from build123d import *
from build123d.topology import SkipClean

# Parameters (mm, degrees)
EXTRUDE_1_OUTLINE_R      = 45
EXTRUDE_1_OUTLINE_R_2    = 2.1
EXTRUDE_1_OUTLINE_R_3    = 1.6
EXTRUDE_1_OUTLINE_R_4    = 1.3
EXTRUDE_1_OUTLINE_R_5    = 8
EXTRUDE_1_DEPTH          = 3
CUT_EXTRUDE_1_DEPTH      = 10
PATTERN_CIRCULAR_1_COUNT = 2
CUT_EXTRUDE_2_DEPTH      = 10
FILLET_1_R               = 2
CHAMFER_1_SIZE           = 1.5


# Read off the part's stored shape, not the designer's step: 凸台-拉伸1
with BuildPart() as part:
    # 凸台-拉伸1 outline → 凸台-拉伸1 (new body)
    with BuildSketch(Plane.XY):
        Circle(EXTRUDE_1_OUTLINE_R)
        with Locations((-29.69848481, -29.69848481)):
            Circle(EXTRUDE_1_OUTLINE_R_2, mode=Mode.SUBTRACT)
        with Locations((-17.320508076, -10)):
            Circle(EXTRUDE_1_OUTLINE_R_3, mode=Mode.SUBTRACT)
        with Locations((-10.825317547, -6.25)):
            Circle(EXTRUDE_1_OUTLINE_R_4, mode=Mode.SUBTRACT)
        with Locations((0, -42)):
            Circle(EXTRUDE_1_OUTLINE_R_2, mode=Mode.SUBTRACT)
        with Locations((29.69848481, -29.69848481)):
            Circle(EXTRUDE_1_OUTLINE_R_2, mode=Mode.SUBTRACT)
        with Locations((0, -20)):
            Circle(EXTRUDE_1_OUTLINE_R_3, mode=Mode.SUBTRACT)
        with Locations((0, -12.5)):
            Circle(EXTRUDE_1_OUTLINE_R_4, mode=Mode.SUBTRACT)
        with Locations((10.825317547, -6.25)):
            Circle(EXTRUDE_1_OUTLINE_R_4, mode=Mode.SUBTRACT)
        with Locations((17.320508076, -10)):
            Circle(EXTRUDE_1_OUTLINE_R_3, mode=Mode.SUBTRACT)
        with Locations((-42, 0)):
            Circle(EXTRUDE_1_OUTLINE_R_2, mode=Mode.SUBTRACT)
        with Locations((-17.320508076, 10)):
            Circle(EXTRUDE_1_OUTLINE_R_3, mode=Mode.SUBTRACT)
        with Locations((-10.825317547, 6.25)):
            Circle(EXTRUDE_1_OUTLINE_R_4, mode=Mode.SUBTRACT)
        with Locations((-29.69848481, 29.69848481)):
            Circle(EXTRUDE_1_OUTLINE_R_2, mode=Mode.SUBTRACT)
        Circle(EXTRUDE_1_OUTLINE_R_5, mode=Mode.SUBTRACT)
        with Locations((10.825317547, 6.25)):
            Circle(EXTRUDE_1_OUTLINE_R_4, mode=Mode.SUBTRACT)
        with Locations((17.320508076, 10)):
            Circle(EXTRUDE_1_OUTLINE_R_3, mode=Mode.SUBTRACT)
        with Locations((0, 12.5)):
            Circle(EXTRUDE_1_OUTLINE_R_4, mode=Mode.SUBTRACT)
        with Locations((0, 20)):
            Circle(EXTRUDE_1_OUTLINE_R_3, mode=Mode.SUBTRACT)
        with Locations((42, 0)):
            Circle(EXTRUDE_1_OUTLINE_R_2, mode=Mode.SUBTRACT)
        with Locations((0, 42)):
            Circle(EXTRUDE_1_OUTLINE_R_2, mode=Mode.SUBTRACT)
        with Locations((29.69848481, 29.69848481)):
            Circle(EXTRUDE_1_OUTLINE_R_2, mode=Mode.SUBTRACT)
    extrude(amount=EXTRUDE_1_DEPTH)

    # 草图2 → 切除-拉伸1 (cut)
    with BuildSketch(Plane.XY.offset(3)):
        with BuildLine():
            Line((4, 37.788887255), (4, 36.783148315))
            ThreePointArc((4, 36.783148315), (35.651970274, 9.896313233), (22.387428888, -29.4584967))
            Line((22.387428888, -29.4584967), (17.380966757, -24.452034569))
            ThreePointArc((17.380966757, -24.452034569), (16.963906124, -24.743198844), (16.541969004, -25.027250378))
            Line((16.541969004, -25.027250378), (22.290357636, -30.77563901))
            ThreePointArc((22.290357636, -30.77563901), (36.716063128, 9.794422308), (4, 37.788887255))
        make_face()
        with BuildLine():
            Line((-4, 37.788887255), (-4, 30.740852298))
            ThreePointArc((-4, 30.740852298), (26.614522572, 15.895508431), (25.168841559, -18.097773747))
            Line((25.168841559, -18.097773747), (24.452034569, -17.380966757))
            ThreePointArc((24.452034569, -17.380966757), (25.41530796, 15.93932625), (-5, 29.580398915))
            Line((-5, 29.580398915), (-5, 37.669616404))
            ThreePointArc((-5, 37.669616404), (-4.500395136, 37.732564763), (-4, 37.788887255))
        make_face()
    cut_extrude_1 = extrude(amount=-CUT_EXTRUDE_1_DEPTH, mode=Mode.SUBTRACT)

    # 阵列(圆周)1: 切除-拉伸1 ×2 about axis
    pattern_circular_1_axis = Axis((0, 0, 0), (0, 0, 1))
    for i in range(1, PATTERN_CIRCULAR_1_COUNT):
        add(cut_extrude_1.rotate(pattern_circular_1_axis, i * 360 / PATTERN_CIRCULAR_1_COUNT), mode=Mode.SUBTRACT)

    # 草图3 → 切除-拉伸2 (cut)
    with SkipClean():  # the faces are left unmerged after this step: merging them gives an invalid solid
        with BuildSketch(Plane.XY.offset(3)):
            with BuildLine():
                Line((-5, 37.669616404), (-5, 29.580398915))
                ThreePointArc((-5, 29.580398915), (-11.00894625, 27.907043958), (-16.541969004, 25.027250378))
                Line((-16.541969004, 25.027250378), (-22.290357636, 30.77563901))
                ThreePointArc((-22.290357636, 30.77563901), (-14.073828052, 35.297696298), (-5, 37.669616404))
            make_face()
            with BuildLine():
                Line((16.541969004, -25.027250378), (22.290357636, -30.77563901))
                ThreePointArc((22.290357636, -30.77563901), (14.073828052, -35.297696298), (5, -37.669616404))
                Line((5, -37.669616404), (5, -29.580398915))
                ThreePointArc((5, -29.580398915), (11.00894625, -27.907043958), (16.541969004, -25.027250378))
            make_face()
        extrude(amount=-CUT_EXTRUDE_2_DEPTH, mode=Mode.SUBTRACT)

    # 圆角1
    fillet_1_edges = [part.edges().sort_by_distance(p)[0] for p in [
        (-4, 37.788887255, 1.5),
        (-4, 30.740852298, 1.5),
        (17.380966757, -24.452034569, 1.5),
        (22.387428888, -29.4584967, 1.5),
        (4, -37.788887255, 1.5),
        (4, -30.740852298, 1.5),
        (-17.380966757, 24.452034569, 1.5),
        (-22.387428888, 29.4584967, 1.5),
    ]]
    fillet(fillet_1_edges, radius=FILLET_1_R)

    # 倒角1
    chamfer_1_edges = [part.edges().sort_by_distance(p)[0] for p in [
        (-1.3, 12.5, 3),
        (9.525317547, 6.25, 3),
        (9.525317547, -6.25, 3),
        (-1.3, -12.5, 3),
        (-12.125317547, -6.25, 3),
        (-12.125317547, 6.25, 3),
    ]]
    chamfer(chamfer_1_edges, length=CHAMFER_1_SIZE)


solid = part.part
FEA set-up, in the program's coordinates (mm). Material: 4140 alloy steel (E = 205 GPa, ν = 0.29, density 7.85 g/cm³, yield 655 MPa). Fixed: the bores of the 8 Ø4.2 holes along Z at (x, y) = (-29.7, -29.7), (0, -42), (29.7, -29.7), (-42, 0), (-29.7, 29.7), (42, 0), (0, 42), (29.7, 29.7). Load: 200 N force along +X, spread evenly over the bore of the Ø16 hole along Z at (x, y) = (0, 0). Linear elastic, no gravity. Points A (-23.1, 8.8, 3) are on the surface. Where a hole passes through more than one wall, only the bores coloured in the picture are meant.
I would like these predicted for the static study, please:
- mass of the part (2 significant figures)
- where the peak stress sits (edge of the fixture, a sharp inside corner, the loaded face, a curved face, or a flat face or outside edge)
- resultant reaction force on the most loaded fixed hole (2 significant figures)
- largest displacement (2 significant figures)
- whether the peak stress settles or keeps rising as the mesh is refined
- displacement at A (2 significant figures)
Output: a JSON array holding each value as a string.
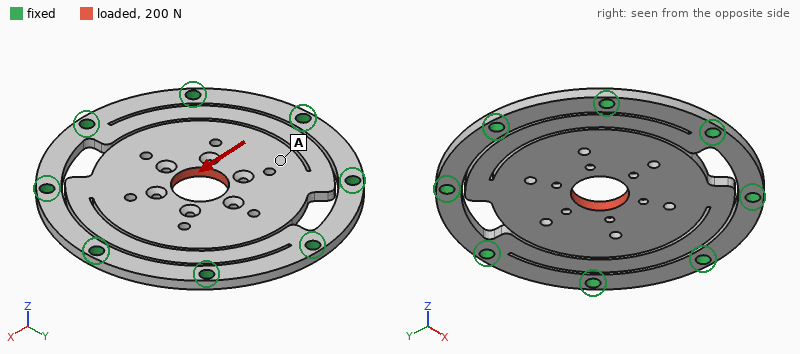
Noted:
["130 g", "a sharp inside corner", "140 N", "0.28 mm", "keeps rising", "0.28 mm"]
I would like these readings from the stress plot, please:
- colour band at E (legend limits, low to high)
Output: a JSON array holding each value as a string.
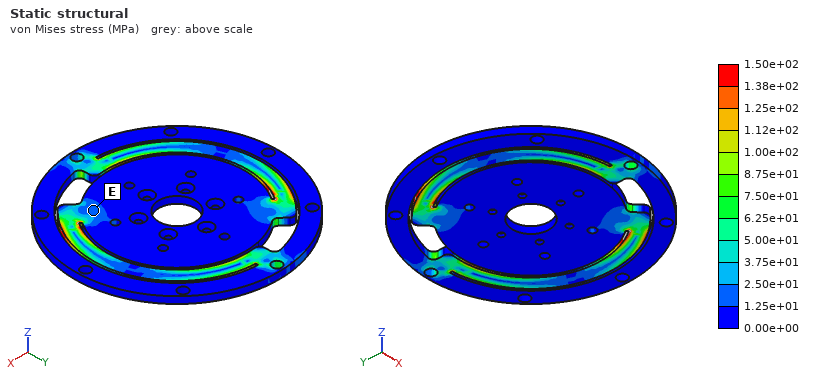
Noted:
["1.25e+01 to 2.50e+01 MPa"]
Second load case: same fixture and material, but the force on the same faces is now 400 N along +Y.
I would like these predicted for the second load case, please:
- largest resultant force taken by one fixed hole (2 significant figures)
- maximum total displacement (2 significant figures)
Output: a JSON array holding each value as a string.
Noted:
["230 N", "0.25 mm"]
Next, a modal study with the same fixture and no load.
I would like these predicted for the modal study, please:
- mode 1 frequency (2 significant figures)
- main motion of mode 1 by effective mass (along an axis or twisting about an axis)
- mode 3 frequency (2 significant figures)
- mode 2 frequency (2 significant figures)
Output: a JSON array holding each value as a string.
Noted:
["230 Hz", "along Z", "480 Hz", "270 Hz"]
